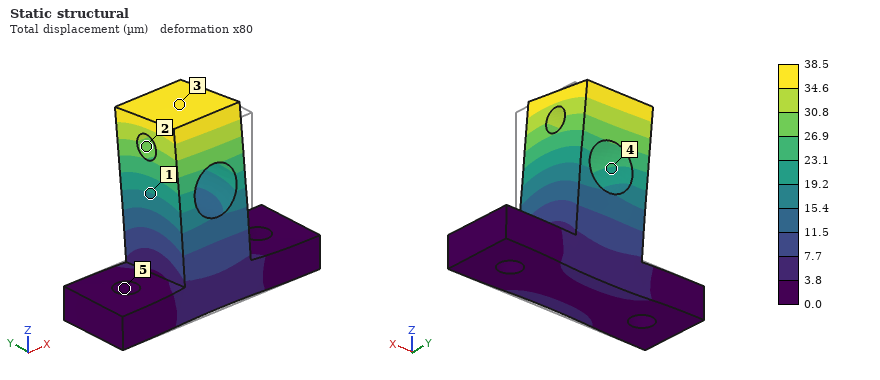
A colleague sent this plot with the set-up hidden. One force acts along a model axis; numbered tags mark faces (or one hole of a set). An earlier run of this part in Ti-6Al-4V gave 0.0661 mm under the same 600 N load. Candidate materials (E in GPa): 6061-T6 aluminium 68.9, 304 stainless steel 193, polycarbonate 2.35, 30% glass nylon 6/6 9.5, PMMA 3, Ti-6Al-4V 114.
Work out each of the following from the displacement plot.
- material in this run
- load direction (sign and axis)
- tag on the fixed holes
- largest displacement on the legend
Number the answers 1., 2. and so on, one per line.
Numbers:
1. 304 stainless steel
2. +Y
3. 5
4. 38.5 µm
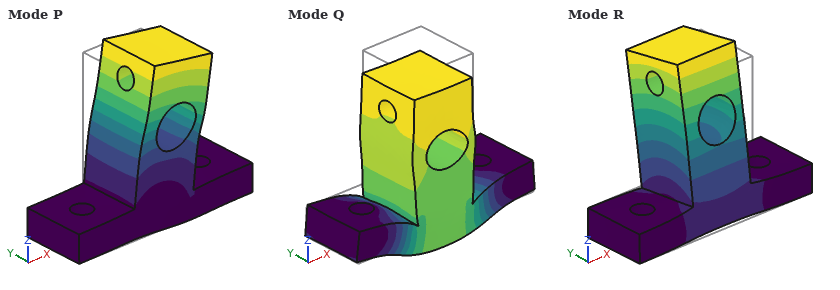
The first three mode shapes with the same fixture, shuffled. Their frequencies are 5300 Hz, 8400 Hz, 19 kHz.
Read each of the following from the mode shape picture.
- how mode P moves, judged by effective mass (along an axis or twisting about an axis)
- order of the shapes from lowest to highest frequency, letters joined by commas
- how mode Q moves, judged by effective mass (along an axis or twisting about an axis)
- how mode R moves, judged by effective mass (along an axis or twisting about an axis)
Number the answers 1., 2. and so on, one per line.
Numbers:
1. along X
2. R, P, Q
3. along Z
4. along Y
